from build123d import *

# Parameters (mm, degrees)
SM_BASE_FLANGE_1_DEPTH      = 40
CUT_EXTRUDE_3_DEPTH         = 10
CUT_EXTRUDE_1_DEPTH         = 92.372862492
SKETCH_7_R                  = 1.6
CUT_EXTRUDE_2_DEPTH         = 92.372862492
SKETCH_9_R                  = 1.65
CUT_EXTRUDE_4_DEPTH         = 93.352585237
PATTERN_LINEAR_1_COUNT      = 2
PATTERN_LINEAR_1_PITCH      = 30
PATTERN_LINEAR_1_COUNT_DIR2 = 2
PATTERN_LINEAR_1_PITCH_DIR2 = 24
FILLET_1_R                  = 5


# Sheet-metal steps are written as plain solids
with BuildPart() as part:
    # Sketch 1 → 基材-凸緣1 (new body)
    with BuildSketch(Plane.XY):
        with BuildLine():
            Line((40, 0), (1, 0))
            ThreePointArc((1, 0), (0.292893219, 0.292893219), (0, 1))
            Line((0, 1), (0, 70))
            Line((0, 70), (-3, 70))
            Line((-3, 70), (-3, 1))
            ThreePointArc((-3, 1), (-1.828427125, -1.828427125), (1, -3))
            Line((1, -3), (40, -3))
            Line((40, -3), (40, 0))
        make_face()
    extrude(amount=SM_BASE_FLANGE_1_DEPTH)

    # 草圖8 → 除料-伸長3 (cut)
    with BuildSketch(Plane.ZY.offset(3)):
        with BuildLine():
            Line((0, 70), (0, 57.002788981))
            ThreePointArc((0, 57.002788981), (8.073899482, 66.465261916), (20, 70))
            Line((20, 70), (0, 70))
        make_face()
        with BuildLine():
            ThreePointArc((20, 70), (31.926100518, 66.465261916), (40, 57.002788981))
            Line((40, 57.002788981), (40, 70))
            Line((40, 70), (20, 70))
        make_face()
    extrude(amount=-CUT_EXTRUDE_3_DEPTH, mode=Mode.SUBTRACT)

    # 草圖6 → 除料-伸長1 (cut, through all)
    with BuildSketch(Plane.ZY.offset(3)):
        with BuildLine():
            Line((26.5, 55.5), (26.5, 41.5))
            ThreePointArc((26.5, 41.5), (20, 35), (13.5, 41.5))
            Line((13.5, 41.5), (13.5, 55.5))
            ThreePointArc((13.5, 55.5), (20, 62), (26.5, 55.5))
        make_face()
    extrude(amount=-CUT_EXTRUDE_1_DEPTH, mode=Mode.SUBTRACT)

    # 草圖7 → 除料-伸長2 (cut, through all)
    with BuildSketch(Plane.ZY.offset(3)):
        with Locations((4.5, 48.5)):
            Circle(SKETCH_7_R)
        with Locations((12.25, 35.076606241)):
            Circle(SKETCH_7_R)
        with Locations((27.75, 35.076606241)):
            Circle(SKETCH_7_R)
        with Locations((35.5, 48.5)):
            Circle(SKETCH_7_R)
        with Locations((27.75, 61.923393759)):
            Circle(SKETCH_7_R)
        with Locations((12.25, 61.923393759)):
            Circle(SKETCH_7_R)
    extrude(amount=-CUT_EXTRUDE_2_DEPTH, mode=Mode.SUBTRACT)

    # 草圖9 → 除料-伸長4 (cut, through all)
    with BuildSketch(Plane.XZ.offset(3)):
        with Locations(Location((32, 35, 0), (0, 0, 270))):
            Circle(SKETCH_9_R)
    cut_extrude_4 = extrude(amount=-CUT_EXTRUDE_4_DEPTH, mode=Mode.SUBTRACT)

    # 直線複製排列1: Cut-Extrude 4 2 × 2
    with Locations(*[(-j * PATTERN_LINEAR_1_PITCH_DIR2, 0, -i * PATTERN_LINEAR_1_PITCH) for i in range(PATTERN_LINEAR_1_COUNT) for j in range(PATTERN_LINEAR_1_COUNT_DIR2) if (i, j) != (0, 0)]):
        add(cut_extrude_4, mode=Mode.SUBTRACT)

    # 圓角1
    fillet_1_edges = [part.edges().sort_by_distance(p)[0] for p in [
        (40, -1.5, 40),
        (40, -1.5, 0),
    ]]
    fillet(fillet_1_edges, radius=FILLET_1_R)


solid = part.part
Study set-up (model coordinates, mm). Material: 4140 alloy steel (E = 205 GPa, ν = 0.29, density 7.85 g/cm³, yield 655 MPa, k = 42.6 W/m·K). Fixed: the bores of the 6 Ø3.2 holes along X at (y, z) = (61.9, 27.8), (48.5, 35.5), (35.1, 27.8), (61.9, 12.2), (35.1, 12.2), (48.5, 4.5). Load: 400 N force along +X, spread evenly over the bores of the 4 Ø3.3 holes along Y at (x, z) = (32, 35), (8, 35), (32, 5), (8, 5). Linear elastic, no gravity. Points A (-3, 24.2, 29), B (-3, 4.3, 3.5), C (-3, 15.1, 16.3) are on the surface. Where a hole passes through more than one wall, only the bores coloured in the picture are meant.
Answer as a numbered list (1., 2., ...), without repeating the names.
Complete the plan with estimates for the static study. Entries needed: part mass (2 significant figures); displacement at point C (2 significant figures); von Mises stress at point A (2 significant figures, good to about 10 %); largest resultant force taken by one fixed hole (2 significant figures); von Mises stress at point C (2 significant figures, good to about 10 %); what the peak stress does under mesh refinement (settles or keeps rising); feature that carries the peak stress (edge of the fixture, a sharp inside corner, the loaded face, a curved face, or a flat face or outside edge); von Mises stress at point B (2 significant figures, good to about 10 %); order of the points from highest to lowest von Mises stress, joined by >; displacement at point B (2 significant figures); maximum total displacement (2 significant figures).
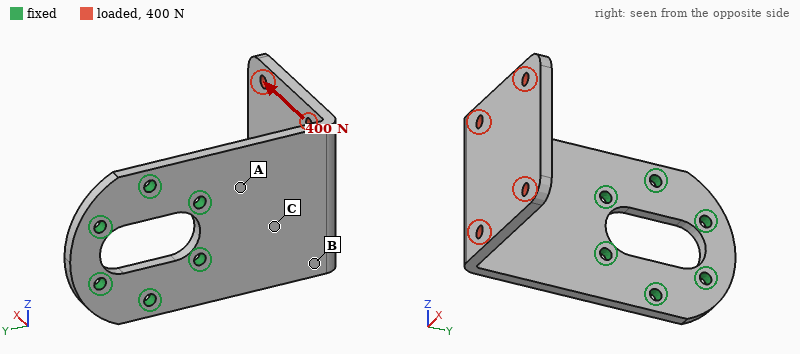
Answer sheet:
1. 92 g
2. 0.14 mm
3. 150 MPa
4. 370 N
5. 98 MPa
6. keeps rising
7. edge of the fixture
8. 41 MPa
9. A > C > B
10. 0.27 mm
11. 0.70 mm
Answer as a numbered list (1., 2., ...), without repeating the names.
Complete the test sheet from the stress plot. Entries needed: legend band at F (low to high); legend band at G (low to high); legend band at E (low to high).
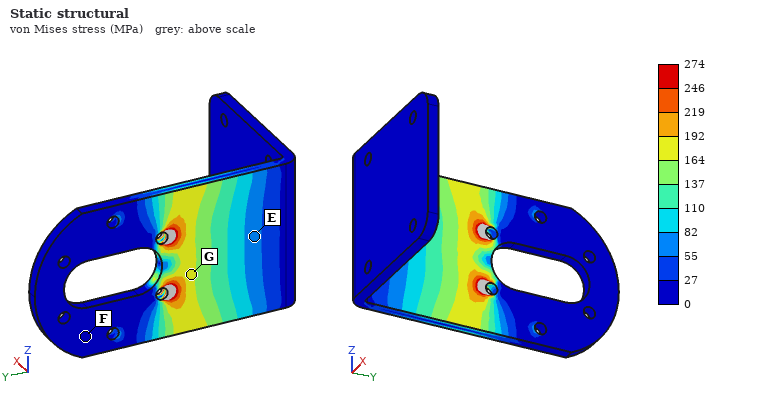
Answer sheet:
1. 0 to 27 MPa
2. 164 to 192 MPa
3. 55 to 82 MPa
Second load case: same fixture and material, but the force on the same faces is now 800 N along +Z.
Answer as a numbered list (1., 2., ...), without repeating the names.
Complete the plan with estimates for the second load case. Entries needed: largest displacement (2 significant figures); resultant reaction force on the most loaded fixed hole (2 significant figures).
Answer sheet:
1. 0.73 mm
2. 1.2 kN
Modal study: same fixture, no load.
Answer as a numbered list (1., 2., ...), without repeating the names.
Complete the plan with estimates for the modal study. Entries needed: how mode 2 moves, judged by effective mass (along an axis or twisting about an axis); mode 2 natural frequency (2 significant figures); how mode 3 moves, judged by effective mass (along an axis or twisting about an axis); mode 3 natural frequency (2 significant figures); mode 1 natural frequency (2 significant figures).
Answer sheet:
1. along Z
2. 980 Hz
3. along X
4. 1500 Hz
5. 560 Hz
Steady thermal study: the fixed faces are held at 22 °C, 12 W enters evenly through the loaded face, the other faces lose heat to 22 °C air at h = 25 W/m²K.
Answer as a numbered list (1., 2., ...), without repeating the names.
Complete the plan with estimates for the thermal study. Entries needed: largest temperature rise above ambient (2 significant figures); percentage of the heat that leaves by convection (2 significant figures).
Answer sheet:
1. 75 K
2. 58 %
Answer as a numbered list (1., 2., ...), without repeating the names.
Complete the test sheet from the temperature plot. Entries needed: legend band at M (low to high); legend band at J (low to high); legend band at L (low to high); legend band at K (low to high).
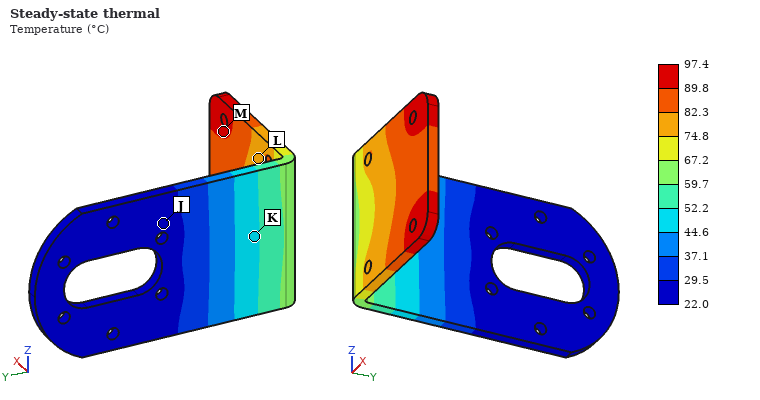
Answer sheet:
1. 89.8 to 97.4 °C
2. 22.0 to 29.5 °C
3. 74.8 to 82.3 °C
4. 44.6 to 52.2 °C
